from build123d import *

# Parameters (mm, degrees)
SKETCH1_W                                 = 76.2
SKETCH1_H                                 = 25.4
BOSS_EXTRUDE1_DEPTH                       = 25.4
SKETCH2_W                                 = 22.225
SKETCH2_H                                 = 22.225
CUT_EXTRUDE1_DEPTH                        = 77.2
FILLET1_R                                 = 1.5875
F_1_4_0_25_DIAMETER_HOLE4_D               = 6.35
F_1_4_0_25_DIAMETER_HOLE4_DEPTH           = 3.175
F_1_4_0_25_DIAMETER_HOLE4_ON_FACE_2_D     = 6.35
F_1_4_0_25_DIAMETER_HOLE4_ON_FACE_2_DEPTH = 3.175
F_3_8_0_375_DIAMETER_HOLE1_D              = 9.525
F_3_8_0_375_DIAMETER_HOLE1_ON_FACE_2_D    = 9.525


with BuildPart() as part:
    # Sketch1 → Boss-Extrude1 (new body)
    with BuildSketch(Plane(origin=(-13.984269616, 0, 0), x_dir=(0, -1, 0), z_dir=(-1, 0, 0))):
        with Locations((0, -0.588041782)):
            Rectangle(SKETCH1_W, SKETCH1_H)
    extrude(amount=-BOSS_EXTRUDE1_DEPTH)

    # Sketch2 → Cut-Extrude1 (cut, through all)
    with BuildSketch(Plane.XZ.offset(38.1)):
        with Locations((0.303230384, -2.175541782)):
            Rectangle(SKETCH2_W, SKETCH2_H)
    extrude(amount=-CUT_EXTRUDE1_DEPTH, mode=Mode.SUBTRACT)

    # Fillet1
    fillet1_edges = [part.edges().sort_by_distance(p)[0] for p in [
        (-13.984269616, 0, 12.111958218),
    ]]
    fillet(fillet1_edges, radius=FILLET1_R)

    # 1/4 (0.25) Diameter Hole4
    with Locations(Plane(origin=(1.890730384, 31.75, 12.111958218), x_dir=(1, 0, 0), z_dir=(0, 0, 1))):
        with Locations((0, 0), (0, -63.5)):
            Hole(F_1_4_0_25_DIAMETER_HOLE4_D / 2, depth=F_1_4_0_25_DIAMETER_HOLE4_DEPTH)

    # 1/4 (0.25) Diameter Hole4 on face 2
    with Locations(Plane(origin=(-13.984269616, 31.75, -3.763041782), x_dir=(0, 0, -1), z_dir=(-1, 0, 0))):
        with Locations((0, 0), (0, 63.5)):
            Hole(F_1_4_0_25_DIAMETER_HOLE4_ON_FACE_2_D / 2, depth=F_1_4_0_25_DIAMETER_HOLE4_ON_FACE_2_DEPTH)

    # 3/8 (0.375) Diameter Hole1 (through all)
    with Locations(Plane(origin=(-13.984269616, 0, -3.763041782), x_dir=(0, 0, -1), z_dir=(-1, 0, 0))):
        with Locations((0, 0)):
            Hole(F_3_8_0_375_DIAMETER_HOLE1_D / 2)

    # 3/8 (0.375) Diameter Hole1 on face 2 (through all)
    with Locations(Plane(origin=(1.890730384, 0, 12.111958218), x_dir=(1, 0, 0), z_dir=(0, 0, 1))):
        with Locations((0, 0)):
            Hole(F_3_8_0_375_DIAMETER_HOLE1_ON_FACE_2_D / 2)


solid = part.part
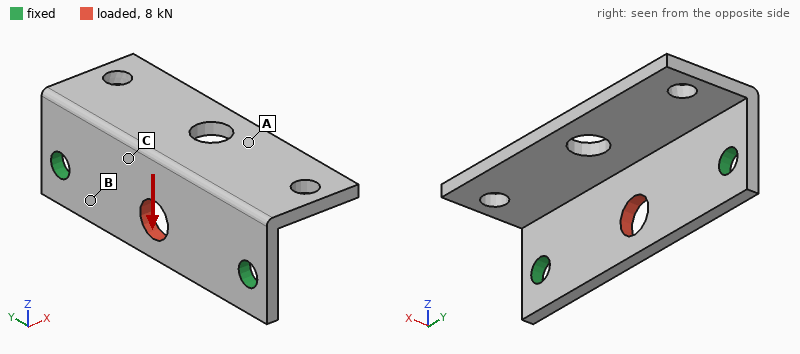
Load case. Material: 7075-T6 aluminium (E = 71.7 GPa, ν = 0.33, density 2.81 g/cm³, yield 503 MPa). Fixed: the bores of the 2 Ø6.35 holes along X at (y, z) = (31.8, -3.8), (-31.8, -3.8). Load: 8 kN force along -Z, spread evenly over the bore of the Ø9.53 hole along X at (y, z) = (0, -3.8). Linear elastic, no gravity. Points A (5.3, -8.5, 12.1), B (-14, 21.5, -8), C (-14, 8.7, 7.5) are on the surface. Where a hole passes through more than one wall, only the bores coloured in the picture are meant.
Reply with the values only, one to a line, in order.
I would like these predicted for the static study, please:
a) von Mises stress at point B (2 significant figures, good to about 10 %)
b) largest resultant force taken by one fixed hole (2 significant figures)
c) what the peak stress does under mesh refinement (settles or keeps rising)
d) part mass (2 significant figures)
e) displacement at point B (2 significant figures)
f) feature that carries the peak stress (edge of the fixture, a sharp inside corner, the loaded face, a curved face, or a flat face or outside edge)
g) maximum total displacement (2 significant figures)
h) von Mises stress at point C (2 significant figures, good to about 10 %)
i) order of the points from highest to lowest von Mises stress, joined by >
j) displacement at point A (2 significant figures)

70 MPa
4.5 kN
keeps rising
30 g
0.042 mm
edge of the fixture
0.13 mm
130 MPa
C > B > A
0.11 mm
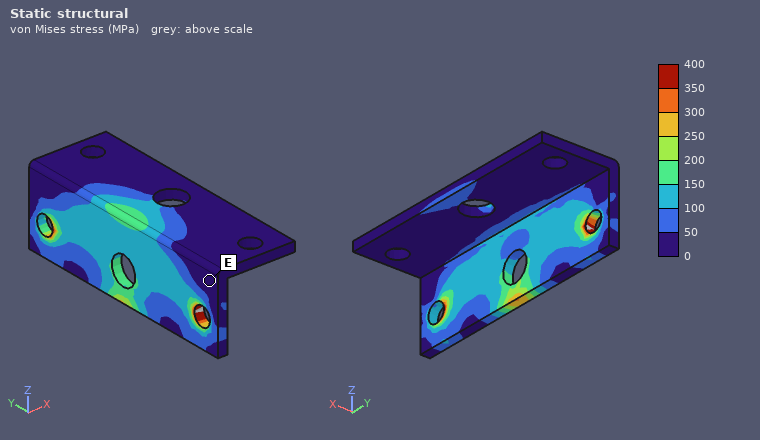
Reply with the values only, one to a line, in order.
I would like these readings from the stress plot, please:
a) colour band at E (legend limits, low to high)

0 to 50 MPa
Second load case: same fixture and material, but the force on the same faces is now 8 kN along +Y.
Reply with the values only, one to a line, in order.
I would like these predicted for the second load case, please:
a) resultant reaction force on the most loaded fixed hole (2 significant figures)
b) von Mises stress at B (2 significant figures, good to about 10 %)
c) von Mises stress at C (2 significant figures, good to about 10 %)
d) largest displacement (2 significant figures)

4.0 kN
75 MPa
19 MPa
31 µm
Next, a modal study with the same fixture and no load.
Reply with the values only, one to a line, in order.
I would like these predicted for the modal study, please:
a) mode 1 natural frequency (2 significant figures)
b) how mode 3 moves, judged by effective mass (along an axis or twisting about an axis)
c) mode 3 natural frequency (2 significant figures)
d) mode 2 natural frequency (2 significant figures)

2200 Hz
along X
5300 Hz
3700 Hz
